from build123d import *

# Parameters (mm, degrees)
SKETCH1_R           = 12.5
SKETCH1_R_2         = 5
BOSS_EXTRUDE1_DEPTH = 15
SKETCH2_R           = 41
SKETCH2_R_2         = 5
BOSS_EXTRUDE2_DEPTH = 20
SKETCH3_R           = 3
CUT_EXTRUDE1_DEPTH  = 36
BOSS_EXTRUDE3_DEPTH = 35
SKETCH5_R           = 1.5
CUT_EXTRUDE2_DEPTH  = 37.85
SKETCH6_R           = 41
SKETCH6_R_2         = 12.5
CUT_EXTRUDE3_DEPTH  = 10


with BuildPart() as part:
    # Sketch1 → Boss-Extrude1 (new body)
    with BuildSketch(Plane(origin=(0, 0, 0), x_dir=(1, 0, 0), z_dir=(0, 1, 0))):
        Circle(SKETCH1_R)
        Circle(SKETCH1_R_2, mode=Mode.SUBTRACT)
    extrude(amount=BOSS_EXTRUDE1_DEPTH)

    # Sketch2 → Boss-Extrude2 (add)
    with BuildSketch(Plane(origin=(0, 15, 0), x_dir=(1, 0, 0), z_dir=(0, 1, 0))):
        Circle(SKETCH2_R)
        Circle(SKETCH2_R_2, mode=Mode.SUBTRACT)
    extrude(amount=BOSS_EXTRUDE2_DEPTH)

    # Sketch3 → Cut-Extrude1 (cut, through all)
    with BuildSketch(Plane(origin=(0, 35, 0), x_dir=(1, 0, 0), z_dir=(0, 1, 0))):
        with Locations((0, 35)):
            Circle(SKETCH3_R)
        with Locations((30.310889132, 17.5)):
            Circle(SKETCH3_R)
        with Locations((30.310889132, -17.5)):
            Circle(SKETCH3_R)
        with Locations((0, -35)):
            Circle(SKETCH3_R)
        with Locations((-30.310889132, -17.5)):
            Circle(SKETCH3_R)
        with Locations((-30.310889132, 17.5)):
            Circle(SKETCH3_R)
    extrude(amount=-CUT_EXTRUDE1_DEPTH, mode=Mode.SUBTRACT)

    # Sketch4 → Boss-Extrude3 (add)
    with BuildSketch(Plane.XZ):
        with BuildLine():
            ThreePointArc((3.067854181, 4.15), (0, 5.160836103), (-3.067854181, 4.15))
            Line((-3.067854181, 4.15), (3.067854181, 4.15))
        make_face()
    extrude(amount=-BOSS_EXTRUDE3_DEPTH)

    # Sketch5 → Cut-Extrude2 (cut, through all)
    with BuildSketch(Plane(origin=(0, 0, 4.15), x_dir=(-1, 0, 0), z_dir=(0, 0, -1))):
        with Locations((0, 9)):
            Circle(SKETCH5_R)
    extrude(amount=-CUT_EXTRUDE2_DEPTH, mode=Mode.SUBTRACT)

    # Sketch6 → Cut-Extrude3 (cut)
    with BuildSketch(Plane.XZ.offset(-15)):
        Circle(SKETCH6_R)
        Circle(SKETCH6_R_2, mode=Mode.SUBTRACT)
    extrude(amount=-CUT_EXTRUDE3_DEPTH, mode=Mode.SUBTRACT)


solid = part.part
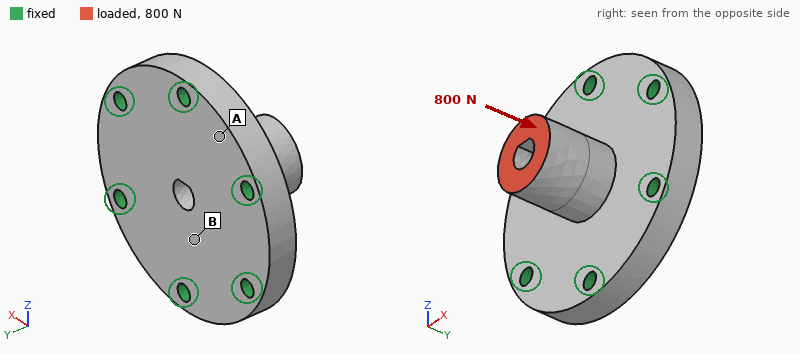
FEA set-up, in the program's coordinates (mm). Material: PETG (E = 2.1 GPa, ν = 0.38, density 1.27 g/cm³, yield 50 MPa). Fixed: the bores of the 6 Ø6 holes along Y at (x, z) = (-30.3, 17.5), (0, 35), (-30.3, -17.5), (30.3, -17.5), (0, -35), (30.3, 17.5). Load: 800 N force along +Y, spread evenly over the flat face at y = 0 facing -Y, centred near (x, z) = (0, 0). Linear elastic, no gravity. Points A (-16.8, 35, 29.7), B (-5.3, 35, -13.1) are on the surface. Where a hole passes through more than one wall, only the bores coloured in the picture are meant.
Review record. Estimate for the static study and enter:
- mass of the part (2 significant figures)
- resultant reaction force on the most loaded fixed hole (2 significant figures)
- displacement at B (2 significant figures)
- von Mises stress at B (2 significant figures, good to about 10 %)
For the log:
77 g
140 N
0.066 mm
2.8 MPa
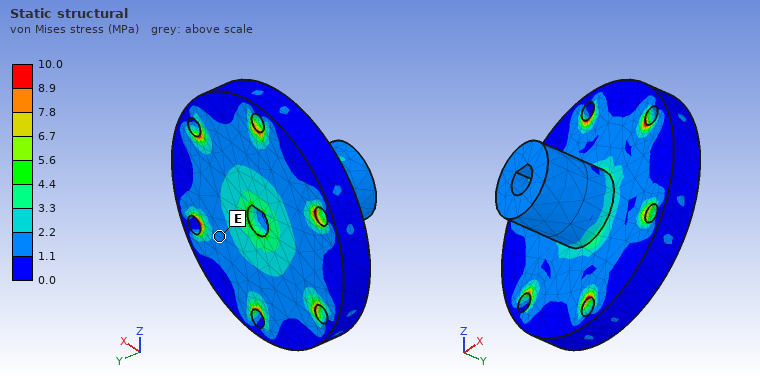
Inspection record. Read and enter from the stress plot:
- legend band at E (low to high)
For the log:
1.1 to 2.2 MPa
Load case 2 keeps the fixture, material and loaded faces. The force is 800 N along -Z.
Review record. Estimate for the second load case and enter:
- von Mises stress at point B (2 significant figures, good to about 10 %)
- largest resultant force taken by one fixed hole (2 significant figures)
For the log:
6.7 MPa
360 N
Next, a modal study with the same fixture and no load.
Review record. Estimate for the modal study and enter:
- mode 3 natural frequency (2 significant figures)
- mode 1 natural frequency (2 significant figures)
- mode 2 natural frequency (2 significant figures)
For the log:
3000 Hz
2900 Hz
2900 Hz
